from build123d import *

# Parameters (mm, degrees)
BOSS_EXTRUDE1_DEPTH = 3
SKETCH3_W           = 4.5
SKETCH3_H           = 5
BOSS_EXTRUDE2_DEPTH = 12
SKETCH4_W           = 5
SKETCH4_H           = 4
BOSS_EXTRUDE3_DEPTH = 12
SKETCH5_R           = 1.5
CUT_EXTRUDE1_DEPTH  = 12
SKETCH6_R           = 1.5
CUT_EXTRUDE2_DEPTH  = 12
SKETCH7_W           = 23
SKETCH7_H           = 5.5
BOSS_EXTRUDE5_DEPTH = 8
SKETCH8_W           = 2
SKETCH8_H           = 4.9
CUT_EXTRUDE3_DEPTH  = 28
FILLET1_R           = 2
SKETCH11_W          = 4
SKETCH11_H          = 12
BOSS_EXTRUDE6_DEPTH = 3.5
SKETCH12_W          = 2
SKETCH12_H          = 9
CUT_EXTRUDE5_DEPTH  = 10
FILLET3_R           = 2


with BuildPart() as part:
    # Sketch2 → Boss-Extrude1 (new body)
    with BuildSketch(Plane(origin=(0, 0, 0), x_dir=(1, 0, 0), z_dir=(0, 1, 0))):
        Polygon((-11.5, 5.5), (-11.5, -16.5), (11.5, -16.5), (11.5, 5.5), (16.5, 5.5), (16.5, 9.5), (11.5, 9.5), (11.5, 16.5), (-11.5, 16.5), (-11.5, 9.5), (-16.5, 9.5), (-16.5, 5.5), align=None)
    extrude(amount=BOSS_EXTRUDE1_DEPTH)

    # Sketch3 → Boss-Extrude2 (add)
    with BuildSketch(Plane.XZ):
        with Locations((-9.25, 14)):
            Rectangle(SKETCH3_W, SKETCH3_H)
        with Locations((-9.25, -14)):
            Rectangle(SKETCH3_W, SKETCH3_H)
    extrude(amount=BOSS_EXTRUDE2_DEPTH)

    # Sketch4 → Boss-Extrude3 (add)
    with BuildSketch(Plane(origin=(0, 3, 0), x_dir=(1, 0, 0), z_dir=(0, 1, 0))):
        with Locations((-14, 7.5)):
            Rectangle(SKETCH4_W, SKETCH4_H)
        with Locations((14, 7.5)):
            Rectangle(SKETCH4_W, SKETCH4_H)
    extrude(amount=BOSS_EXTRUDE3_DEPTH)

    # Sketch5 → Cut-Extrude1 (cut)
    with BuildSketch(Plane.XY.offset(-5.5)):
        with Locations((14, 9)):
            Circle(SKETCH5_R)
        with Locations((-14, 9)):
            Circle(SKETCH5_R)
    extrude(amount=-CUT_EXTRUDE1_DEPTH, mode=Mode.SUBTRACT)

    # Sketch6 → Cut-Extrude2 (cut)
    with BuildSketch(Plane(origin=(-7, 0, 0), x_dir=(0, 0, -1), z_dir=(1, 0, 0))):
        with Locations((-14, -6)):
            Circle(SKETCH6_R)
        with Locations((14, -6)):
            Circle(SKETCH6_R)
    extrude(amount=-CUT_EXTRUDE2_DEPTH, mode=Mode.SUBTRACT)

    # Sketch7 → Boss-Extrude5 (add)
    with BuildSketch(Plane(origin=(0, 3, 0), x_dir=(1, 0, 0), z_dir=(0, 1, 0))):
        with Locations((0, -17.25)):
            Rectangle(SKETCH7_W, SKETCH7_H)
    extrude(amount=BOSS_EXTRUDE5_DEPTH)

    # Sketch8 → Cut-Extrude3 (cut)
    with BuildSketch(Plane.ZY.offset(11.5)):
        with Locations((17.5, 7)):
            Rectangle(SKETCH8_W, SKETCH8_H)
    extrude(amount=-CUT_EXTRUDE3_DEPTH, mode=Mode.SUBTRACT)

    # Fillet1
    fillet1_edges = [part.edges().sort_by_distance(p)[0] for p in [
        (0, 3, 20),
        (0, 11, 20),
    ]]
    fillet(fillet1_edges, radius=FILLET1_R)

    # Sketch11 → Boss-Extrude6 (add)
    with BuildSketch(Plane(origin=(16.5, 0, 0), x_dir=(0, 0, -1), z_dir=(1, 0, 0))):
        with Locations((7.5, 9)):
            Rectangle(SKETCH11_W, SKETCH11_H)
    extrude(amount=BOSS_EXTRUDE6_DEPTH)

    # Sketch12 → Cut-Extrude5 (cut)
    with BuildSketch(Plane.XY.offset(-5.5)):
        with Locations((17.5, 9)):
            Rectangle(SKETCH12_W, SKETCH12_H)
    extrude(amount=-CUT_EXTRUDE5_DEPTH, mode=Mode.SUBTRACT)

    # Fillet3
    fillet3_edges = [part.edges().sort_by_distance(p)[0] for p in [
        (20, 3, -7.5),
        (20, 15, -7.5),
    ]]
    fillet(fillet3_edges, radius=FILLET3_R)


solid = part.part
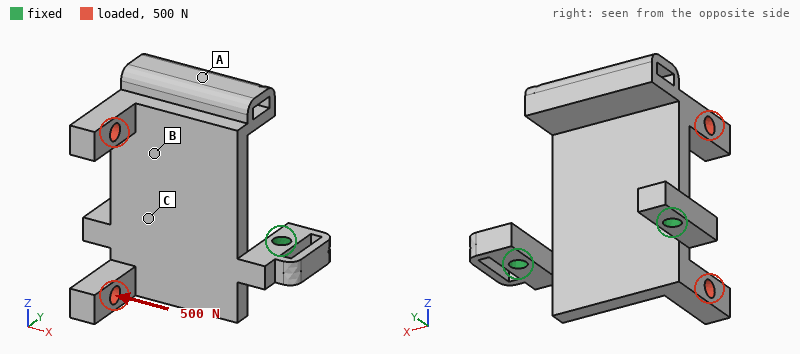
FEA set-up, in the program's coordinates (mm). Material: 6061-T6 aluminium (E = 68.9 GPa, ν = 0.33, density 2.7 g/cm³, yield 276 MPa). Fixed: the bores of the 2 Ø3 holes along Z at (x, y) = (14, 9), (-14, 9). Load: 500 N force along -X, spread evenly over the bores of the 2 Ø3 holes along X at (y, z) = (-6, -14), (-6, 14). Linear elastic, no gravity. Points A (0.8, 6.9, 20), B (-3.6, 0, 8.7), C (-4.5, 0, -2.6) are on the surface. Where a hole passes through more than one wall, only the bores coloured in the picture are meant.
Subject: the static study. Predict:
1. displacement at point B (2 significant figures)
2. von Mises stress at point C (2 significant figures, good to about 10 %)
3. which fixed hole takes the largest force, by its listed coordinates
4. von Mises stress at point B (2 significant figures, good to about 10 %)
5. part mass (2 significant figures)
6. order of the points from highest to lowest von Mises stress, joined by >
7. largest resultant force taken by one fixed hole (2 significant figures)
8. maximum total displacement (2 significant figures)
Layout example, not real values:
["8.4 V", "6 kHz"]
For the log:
["0.029 mm", "25 MPa", "(14, 9)", "46 MPa", "11 g", "B > C > A", "380 N", "0.16 mm"]
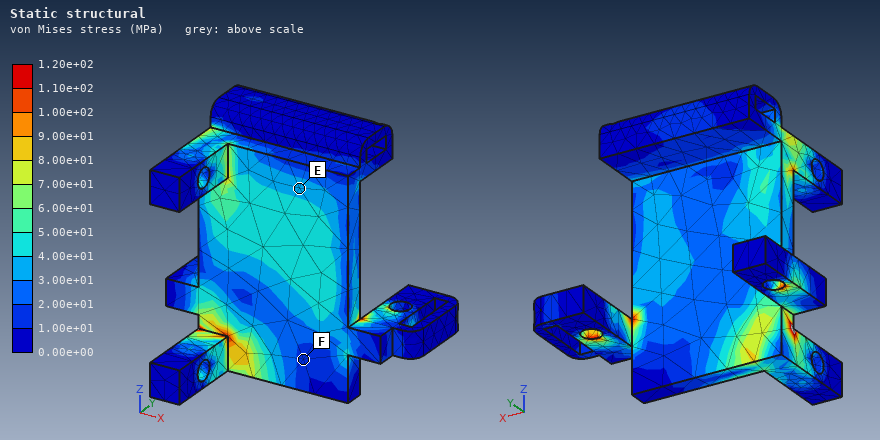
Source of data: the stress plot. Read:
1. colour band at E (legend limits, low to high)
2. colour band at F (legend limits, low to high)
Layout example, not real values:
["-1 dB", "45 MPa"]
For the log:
["3.00e+01 to 4.00e+01 MPa", "1.00e+01 to 2.00e+01 MPa"]
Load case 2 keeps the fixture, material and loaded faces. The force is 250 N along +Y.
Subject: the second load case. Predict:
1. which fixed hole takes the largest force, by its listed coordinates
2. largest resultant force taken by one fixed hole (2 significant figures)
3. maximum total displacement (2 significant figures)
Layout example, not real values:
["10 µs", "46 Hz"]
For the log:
["(-14, 9)", "240 N", "0.40 mm"]
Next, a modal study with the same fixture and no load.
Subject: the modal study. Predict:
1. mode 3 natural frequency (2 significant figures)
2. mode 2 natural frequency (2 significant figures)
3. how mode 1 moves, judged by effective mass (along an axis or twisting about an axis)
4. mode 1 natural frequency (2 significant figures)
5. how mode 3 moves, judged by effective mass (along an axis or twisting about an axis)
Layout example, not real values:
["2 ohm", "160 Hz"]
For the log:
["6200 Hz", "4400 Hz", "along Y", "1400 Hz", "along Z"]
